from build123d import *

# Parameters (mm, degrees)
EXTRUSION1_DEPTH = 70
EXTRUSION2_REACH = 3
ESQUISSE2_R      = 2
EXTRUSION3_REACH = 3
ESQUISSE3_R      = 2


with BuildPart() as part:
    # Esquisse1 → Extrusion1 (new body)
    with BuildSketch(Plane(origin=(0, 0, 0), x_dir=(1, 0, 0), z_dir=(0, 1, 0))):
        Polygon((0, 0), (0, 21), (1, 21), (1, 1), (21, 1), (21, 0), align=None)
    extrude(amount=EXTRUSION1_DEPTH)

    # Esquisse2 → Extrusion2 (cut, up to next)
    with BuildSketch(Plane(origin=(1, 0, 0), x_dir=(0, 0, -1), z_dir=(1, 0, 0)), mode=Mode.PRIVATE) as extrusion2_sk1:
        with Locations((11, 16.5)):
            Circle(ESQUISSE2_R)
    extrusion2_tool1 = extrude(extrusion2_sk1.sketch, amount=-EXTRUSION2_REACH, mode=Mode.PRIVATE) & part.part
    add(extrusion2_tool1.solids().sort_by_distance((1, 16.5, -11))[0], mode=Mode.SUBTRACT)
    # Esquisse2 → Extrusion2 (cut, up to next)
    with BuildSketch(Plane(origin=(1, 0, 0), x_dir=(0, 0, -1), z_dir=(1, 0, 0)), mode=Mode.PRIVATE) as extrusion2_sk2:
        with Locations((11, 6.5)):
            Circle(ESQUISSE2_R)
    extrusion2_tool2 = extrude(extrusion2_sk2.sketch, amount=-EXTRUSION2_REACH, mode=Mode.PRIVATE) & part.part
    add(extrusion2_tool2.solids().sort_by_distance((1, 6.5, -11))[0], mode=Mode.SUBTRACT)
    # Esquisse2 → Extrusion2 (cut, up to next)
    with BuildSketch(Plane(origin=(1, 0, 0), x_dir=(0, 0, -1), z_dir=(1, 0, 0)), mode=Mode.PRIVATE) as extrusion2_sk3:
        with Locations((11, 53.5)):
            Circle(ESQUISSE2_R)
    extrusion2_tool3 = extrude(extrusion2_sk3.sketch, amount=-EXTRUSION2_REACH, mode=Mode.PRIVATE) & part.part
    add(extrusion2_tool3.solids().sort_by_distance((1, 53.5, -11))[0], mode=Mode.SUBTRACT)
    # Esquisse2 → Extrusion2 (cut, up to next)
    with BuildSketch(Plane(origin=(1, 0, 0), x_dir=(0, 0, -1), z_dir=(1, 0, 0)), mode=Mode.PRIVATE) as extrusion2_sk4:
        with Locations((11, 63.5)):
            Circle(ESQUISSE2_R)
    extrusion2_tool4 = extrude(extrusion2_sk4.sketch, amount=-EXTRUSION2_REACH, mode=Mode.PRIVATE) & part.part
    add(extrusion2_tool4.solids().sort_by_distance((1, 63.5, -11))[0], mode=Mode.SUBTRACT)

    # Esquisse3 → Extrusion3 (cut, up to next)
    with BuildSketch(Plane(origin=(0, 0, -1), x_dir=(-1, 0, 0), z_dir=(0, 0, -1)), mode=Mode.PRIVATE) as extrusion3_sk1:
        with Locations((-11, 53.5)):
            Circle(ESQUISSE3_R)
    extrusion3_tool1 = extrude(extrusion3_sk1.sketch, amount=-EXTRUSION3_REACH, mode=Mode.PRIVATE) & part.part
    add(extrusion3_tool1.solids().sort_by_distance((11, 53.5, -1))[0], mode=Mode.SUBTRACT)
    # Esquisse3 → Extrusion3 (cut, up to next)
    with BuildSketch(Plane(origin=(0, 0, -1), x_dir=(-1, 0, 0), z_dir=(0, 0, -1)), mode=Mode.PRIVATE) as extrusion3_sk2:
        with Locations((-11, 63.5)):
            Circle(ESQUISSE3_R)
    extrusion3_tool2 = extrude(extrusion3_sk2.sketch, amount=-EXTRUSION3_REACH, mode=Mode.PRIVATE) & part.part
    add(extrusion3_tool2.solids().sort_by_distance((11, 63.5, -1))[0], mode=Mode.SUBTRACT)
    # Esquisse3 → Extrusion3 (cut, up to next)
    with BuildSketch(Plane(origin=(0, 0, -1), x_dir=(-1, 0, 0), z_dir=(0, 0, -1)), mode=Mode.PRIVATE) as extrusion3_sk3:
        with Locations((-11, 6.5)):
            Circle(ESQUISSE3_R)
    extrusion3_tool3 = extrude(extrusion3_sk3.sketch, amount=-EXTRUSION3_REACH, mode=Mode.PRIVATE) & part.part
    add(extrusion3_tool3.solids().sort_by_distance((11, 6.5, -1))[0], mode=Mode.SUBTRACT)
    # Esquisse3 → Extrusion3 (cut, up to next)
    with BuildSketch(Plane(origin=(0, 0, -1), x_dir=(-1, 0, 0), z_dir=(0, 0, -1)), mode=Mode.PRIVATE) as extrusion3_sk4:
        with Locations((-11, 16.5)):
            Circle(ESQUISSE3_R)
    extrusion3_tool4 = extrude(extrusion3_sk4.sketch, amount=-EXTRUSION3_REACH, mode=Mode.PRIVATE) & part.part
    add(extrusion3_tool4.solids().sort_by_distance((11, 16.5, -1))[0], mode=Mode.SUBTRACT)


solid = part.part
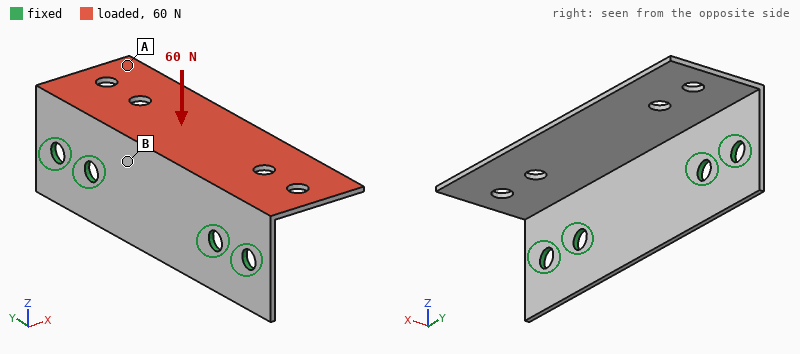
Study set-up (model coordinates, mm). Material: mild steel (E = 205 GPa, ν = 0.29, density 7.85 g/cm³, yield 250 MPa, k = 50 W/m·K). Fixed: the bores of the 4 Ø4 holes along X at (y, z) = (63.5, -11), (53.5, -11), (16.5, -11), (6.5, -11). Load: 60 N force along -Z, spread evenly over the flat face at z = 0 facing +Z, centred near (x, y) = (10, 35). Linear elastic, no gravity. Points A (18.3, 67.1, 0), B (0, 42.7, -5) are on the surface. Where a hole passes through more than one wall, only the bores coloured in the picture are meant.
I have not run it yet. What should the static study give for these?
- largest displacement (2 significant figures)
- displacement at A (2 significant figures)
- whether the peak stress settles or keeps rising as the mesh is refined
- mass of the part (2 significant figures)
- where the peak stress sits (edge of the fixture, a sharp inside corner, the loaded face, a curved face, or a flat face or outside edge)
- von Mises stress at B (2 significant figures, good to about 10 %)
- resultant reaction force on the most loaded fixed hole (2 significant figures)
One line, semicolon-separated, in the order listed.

0.15 mm; 0.13 mm; keeps rising; 22 g; edge of the fixture; 35 MPa; 26 N
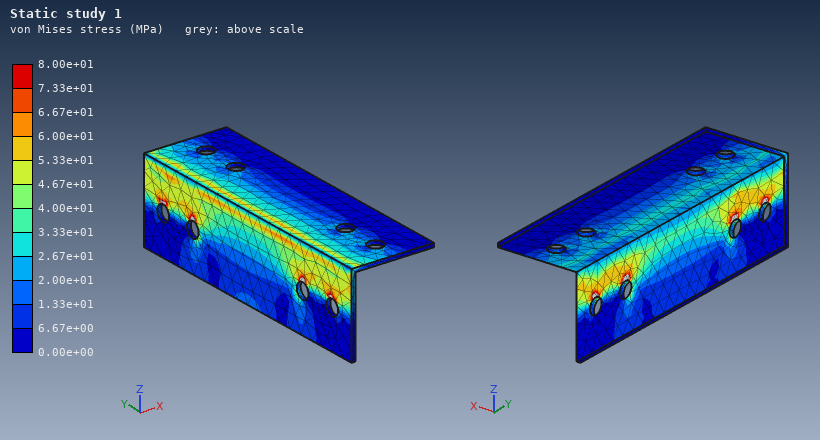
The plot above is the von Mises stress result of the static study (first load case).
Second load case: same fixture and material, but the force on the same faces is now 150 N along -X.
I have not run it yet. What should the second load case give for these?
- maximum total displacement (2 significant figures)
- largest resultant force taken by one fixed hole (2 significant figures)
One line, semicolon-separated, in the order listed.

0.16 mm; 41 N
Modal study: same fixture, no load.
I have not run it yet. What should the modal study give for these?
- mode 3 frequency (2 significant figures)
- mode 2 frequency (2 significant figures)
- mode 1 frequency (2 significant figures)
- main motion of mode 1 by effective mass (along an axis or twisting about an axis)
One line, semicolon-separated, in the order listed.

3100 Hz; 1700 Hz; 1100 Hz; along Z
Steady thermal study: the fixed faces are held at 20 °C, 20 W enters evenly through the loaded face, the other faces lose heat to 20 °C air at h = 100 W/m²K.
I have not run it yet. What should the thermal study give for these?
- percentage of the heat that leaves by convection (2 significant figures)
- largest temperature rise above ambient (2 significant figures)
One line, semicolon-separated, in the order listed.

59 %; 65 K
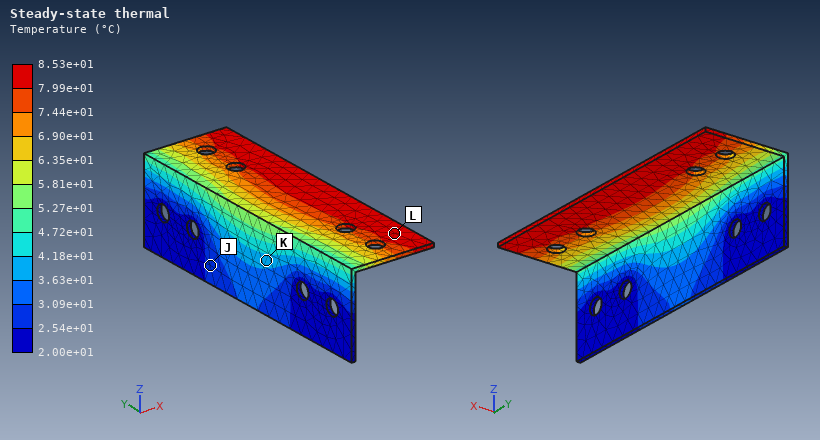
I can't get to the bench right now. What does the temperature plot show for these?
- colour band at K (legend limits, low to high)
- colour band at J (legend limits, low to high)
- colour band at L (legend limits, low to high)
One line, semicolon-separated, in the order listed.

3.63e+01 to 4.18e+01 °C; 2.54e+01 to 3.09e+01 °C; 7.99e+01 to 8.53e+01 °C
